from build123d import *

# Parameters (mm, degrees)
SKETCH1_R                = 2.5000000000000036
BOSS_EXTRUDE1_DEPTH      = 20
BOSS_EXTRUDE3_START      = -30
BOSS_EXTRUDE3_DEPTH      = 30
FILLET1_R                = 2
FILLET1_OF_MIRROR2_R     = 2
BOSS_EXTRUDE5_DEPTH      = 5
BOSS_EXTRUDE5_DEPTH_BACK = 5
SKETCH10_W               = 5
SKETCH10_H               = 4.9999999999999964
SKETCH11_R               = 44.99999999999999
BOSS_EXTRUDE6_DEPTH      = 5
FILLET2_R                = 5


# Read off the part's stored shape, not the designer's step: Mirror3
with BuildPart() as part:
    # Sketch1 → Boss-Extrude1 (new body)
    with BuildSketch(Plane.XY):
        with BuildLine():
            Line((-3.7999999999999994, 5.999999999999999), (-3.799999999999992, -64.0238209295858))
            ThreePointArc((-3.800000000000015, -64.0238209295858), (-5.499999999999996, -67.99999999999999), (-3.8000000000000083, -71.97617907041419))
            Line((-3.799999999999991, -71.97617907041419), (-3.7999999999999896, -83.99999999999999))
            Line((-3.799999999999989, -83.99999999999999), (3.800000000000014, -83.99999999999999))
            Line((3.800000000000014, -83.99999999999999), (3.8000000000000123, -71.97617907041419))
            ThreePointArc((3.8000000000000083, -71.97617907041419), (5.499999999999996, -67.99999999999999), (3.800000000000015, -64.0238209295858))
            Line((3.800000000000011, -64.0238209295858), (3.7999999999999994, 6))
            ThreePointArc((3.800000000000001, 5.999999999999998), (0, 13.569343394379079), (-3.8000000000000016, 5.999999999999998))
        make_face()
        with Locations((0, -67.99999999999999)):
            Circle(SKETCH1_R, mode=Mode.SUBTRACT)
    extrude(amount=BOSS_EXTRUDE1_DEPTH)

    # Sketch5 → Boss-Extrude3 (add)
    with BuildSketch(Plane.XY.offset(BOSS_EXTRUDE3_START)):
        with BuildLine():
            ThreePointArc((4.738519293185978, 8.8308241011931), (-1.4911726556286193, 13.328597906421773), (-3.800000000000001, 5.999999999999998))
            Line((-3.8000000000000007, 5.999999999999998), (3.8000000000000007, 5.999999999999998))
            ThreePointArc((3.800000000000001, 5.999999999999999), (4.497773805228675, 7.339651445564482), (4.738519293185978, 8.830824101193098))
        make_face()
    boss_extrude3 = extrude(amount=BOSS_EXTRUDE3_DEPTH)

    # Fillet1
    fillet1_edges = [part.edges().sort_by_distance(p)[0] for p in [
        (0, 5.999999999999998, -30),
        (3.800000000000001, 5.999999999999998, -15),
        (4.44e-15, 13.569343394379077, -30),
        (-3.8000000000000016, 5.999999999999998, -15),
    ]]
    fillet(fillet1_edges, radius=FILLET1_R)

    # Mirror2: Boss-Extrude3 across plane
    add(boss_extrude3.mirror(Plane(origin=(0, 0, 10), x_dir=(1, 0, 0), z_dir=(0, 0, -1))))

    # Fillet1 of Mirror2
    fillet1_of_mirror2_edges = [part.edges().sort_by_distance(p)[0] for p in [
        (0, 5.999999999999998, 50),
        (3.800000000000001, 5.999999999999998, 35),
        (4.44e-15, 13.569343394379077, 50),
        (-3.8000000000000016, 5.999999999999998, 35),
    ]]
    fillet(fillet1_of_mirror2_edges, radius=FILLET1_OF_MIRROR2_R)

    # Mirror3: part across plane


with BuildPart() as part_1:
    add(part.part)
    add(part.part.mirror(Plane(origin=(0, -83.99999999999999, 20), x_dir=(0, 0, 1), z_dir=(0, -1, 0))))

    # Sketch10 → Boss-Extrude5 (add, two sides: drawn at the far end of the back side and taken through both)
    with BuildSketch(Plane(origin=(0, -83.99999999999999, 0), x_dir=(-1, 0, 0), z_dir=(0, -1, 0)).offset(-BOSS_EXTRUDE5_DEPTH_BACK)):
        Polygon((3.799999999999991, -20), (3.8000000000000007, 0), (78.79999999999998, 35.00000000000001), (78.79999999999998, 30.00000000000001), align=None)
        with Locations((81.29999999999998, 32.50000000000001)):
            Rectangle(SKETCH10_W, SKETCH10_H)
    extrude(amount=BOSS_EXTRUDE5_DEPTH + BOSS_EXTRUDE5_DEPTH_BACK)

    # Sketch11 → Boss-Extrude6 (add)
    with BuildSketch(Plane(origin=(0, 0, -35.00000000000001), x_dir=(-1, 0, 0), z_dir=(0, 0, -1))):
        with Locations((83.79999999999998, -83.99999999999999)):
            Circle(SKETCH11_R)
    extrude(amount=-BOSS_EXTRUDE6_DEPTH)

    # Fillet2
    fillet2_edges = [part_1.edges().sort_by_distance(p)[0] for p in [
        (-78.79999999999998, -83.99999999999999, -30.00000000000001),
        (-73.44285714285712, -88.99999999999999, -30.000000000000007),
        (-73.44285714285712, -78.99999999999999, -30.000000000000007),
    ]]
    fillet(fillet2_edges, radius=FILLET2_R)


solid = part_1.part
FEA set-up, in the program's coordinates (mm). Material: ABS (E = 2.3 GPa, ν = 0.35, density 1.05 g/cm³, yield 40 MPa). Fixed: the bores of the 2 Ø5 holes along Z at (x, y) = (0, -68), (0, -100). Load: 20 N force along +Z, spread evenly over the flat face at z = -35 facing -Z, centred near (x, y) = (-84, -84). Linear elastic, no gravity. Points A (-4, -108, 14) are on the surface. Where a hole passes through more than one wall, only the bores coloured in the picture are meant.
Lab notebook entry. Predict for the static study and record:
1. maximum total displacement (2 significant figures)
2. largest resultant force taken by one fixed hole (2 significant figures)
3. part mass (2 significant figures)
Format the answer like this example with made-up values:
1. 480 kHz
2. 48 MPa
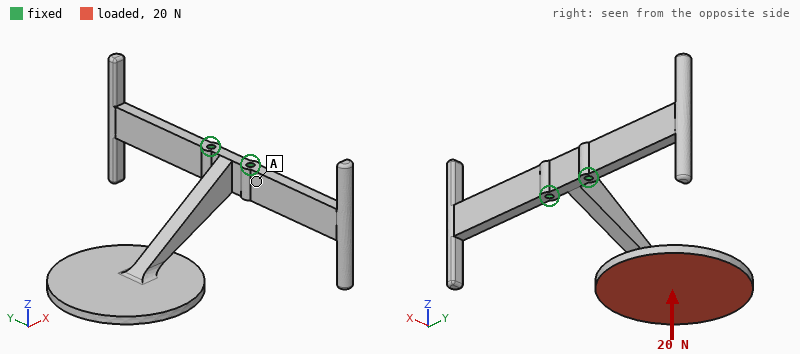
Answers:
1. 2.9 mm
2. 12 N
3. 82 g
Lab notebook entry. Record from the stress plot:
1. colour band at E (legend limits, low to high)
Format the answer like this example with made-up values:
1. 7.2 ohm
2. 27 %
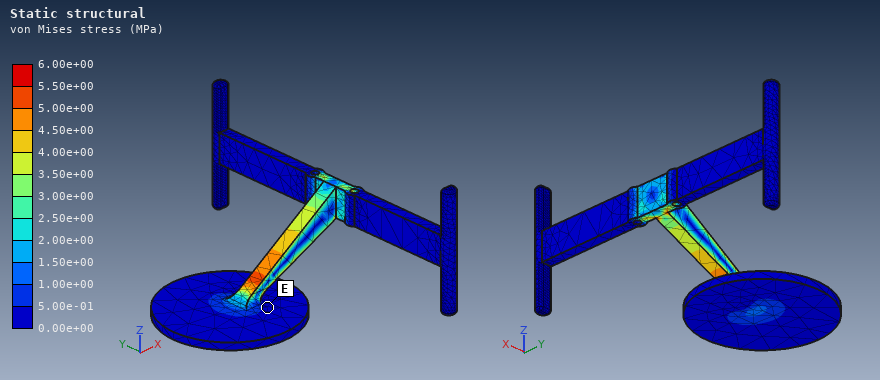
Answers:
1. 0.00e+00 to 5.00e-01 MPa
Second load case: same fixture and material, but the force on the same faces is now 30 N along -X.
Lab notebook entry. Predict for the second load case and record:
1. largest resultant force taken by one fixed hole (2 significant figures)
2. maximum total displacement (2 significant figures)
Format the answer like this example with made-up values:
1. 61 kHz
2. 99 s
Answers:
1. 18 N
2. 2.3 mm
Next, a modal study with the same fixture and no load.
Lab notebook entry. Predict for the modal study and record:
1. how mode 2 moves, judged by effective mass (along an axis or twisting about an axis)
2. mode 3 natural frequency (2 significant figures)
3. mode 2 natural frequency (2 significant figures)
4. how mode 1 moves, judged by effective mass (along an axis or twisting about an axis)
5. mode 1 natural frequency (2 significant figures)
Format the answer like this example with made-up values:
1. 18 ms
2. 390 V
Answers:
1. along Z
2. 140 Hz
3. 86 Hz
4. along Y
5. 74 Hz
